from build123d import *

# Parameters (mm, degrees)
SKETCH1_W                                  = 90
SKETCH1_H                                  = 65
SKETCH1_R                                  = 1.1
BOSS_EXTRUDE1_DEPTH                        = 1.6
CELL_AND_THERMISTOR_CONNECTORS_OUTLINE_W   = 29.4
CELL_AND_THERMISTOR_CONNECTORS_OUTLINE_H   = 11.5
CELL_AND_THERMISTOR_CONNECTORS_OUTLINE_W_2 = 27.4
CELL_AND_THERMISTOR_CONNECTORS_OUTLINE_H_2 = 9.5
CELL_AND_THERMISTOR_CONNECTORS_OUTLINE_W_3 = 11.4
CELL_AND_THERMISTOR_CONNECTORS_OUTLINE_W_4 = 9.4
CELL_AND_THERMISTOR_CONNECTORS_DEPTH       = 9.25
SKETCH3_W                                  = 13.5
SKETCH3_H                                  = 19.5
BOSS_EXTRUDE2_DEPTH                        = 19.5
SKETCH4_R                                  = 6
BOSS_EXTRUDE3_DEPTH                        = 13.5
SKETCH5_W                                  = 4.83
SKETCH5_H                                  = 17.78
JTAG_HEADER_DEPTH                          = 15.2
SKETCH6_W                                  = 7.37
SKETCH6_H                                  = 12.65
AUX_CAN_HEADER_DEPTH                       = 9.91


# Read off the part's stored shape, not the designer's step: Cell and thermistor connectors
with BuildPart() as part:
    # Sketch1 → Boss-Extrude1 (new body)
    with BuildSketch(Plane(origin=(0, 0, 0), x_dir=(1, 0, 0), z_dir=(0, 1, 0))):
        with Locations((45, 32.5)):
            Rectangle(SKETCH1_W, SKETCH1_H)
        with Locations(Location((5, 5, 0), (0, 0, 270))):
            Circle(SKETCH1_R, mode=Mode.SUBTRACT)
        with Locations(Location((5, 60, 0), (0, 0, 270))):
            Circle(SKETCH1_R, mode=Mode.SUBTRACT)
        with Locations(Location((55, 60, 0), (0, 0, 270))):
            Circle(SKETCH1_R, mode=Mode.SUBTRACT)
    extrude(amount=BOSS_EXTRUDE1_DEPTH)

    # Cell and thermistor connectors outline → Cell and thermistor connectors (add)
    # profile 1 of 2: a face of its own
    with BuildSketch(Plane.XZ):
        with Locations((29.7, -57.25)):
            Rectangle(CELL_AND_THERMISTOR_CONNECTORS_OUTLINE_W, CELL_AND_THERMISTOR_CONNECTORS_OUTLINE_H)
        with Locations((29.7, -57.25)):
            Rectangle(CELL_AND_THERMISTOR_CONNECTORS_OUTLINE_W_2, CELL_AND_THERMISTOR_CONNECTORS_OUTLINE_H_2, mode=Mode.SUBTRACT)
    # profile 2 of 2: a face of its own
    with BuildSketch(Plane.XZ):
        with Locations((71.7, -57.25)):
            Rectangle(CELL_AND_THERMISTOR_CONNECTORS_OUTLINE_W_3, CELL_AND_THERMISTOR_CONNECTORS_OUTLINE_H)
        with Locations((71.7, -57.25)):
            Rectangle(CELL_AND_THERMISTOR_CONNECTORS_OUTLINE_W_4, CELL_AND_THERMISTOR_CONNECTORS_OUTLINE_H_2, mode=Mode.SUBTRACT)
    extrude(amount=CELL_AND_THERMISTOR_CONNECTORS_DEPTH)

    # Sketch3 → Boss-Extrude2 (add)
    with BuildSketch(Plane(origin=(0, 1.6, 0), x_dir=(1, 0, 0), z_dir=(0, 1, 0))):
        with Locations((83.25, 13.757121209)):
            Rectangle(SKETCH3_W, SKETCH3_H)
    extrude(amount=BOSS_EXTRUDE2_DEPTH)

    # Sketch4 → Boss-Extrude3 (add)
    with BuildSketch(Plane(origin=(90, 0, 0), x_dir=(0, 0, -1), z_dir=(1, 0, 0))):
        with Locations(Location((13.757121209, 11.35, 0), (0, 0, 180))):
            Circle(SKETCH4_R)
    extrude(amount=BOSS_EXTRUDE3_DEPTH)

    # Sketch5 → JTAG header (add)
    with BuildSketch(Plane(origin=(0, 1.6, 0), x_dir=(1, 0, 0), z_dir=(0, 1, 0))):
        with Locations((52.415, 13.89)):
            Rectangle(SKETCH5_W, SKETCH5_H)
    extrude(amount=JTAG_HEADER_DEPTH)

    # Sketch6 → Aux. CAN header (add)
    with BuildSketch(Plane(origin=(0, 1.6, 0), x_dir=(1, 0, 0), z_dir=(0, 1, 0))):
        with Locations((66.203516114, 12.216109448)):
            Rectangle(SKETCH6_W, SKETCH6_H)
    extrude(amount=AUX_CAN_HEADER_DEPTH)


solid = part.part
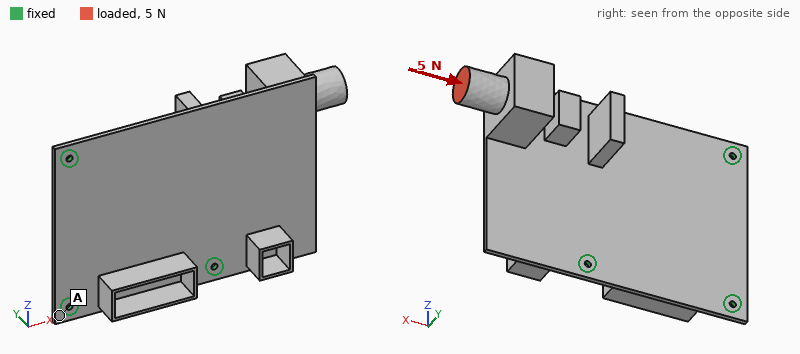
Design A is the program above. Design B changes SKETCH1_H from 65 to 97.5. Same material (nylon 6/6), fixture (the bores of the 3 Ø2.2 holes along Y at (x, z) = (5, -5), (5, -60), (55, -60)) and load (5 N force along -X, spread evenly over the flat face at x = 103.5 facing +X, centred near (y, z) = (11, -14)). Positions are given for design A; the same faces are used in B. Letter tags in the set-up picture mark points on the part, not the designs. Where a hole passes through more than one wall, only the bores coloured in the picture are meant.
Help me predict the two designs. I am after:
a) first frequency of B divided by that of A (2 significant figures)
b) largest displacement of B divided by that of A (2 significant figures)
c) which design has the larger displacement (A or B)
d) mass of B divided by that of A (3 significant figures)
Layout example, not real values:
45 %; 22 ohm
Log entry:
1.1; 0.84; A; 1.24
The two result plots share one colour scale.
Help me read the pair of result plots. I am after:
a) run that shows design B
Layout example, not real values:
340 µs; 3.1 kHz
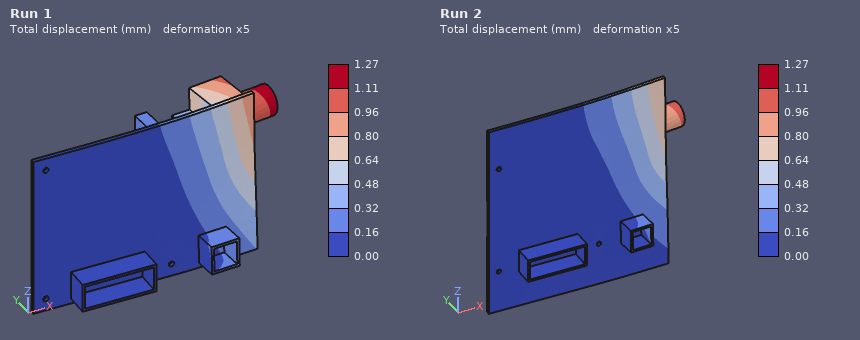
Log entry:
Run 2
